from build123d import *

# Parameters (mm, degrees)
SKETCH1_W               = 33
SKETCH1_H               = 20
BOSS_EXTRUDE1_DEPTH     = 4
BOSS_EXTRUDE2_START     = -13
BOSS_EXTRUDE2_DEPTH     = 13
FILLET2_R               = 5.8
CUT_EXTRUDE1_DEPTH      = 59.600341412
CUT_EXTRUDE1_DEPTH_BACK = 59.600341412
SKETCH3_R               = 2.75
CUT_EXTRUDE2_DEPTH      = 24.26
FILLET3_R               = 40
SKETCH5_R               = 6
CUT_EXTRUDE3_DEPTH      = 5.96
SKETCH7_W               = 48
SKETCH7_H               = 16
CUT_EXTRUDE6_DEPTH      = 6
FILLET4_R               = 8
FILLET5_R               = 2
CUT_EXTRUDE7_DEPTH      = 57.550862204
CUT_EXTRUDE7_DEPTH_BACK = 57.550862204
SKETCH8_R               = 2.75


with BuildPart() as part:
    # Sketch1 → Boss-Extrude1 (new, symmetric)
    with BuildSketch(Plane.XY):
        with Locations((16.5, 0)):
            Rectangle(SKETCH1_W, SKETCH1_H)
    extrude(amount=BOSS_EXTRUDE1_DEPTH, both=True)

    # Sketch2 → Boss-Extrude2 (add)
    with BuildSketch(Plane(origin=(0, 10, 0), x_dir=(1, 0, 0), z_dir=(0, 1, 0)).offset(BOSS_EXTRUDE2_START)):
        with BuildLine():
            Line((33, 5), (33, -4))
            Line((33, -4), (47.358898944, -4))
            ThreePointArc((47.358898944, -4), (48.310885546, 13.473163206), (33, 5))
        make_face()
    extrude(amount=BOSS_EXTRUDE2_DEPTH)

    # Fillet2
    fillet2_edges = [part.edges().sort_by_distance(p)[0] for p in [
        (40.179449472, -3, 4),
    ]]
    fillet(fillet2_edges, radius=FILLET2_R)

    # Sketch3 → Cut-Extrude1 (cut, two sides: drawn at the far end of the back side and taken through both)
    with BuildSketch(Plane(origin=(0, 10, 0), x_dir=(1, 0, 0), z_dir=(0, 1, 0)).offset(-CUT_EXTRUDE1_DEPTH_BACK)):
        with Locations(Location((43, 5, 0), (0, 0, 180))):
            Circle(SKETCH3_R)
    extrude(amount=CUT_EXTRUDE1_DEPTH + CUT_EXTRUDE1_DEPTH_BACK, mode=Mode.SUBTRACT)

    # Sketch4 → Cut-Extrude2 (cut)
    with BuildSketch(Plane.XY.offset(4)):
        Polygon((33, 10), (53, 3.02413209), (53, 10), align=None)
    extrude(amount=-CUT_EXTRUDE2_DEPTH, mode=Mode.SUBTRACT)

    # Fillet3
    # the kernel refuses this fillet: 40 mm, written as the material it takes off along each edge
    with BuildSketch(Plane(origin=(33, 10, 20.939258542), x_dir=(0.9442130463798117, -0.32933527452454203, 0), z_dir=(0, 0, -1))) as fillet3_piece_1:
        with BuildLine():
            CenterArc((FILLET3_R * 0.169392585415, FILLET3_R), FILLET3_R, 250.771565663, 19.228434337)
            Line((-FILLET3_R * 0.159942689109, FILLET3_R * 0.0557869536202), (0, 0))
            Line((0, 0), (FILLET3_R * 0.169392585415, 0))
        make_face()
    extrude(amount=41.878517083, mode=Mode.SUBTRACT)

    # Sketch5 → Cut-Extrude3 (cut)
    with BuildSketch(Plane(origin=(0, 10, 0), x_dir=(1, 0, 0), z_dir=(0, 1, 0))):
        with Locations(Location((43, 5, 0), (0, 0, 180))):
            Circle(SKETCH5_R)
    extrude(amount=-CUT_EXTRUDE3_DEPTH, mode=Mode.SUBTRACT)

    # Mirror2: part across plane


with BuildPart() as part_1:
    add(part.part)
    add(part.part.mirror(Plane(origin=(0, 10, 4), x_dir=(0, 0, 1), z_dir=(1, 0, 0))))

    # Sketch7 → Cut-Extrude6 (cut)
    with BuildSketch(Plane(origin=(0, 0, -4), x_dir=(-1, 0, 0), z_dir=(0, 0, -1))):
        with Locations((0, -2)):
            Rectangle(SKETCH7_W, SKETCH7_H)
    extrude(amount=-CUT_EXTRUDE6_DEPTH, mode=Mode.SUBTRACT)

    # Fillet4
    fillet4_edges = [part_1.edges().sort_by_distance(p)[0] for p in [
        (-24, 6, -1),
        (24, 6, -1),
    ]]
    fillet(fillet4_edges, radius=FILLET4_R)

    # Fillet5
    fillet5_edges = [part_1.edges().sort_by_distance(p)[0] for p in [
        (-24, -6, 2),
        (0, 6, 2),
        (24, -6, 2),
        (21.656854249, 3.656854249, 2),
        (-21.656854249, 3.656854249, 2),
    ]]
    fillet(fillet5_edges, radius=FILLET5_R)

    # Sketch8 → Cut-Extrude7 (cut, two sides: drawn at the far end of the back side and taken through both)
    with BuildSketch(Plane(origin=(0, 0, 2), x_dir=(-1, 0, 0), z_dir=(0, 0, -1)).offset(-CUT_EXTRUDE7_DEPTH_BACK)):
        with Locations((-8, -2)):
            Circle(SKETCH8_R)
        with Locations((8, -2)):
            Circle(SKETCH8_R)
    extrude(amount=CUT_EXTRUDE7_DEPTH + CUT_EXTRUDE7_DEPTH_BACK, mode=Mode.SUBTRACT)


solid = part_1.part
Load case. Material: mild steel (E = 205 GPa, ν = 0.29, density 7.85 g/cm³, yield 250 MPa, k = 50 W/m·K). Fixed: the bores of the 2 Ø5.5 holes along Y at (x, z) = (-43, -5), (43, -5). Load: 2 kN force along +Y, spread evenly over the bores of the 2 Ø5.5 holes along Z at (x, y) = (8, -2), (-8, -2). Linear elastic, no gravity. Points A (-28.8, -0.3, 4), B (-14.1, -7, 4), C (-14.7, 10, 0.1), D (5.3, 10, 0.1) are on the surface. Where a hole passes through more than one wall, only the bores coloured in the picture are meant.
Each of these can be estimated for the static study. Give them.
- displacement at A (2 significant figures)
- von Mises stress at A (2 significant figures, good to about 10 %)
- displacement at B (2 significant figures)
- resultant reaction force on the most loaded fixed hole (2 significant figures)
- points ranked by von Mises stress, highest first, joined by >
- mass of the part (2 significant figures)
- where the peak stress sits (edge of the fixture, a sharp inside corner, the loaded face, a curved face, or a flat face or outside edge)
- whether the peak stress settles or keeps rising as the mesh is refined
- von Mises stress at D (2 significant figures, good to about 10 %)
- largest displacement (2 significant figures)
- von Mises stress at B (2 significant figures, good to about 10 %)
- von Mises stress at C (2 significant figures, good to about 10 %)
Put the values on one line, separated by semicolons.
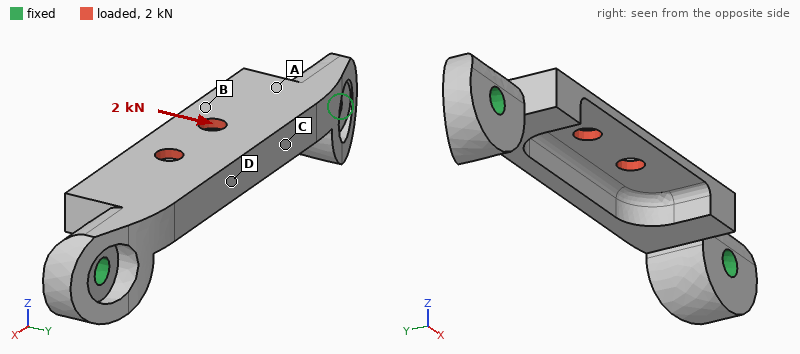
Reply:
13 µm; 31 MPa; 30 µm; 1.2 kN; D > B > C > A; 87 g; edge of the fixture; keeps rising; 81 MPa; 40 µm; 65 MPa; 46 MPa
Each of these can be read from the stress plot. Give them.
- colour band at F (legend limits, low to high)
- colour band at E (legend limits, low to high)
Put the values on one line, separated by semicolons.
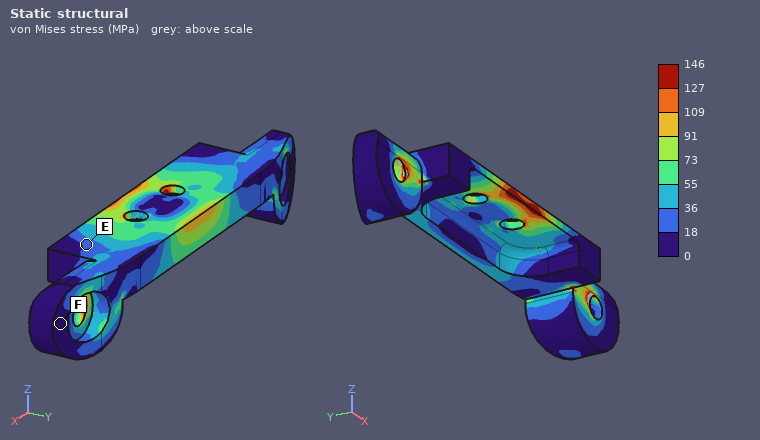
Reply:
0 to 18 MPa; 18 to 36 MPa
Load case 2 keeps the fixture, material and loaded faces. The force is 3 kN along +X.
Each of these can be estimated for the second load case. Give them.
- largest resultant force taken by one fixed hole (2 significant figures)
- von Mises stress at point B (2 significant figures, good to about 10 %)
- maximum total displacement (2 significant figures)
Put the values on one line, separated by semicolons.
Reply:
1.5 kN; 37 MPa; 11 µm
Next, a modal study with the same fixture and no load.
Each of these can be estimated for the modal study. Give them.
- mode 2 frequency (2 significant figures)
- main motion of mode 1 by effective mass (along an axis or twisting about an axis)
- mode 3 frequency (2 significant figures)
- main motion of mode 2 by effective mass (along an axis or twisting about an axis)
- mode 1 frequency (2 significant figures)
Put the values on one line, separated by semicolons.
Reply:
8200 Hz; along Z; 9500 Hz; along Y; 6200 Hz
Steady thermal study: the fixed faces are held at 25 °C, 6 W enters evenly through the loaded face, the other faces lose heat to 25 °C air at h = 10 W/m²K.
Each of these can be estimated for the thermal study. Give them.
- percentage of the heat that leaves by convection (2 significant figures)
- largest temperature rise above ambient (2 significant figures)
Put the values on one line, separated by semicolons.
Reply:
10 %; 32 K
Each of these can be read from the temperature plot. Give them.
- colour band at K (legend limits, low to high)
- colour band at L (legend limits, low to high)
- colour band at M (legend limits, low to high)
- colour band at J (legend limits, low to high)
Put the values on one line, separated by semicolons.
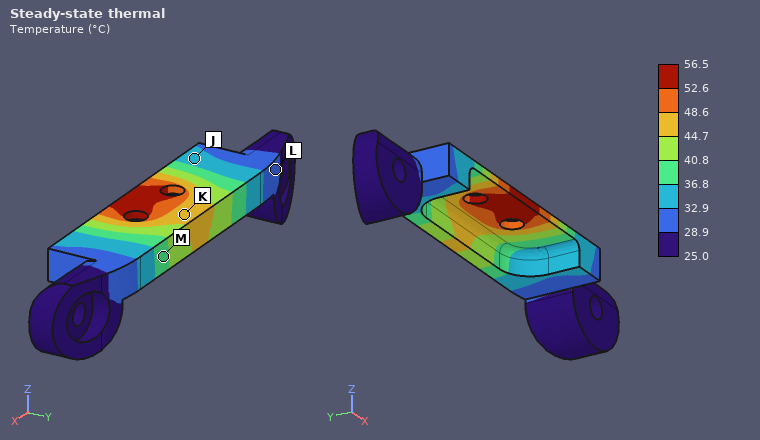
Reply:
44.7 to 48.6 °C; 28.9 to 32.9 °C; 36.8 to 40.8 °C; 32.9 to 36.8 °C
